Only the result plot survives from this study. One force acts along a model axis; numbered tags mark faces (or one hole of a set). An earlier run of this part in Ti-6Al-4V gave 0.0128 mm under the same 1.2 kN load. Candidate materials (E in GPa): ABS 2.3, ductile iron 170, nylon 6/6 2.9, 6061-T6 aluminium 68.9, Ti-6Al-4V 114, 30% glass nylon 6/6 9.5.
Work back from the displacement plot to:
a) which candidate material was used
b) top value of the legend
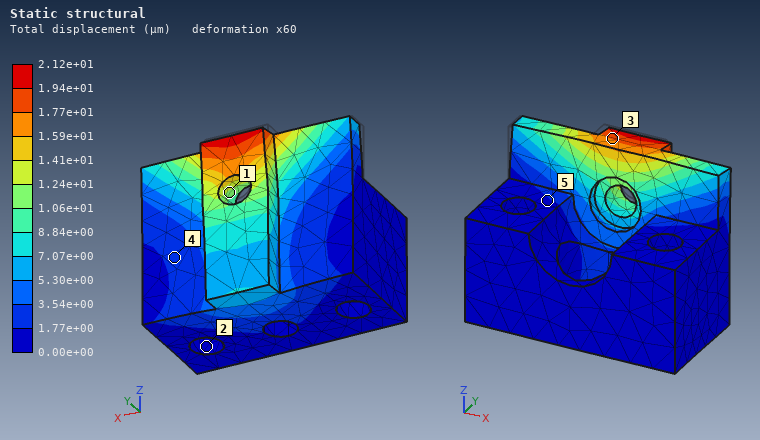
6061-T6 aluminium
2.12e+01 µm
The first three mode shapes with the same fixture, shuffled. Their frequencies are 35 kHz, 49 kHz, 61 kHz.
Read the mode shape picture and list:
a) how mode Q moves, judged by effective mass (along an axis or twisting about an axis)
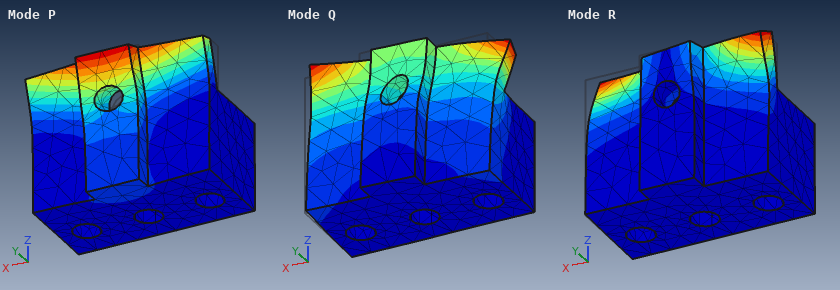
along X
